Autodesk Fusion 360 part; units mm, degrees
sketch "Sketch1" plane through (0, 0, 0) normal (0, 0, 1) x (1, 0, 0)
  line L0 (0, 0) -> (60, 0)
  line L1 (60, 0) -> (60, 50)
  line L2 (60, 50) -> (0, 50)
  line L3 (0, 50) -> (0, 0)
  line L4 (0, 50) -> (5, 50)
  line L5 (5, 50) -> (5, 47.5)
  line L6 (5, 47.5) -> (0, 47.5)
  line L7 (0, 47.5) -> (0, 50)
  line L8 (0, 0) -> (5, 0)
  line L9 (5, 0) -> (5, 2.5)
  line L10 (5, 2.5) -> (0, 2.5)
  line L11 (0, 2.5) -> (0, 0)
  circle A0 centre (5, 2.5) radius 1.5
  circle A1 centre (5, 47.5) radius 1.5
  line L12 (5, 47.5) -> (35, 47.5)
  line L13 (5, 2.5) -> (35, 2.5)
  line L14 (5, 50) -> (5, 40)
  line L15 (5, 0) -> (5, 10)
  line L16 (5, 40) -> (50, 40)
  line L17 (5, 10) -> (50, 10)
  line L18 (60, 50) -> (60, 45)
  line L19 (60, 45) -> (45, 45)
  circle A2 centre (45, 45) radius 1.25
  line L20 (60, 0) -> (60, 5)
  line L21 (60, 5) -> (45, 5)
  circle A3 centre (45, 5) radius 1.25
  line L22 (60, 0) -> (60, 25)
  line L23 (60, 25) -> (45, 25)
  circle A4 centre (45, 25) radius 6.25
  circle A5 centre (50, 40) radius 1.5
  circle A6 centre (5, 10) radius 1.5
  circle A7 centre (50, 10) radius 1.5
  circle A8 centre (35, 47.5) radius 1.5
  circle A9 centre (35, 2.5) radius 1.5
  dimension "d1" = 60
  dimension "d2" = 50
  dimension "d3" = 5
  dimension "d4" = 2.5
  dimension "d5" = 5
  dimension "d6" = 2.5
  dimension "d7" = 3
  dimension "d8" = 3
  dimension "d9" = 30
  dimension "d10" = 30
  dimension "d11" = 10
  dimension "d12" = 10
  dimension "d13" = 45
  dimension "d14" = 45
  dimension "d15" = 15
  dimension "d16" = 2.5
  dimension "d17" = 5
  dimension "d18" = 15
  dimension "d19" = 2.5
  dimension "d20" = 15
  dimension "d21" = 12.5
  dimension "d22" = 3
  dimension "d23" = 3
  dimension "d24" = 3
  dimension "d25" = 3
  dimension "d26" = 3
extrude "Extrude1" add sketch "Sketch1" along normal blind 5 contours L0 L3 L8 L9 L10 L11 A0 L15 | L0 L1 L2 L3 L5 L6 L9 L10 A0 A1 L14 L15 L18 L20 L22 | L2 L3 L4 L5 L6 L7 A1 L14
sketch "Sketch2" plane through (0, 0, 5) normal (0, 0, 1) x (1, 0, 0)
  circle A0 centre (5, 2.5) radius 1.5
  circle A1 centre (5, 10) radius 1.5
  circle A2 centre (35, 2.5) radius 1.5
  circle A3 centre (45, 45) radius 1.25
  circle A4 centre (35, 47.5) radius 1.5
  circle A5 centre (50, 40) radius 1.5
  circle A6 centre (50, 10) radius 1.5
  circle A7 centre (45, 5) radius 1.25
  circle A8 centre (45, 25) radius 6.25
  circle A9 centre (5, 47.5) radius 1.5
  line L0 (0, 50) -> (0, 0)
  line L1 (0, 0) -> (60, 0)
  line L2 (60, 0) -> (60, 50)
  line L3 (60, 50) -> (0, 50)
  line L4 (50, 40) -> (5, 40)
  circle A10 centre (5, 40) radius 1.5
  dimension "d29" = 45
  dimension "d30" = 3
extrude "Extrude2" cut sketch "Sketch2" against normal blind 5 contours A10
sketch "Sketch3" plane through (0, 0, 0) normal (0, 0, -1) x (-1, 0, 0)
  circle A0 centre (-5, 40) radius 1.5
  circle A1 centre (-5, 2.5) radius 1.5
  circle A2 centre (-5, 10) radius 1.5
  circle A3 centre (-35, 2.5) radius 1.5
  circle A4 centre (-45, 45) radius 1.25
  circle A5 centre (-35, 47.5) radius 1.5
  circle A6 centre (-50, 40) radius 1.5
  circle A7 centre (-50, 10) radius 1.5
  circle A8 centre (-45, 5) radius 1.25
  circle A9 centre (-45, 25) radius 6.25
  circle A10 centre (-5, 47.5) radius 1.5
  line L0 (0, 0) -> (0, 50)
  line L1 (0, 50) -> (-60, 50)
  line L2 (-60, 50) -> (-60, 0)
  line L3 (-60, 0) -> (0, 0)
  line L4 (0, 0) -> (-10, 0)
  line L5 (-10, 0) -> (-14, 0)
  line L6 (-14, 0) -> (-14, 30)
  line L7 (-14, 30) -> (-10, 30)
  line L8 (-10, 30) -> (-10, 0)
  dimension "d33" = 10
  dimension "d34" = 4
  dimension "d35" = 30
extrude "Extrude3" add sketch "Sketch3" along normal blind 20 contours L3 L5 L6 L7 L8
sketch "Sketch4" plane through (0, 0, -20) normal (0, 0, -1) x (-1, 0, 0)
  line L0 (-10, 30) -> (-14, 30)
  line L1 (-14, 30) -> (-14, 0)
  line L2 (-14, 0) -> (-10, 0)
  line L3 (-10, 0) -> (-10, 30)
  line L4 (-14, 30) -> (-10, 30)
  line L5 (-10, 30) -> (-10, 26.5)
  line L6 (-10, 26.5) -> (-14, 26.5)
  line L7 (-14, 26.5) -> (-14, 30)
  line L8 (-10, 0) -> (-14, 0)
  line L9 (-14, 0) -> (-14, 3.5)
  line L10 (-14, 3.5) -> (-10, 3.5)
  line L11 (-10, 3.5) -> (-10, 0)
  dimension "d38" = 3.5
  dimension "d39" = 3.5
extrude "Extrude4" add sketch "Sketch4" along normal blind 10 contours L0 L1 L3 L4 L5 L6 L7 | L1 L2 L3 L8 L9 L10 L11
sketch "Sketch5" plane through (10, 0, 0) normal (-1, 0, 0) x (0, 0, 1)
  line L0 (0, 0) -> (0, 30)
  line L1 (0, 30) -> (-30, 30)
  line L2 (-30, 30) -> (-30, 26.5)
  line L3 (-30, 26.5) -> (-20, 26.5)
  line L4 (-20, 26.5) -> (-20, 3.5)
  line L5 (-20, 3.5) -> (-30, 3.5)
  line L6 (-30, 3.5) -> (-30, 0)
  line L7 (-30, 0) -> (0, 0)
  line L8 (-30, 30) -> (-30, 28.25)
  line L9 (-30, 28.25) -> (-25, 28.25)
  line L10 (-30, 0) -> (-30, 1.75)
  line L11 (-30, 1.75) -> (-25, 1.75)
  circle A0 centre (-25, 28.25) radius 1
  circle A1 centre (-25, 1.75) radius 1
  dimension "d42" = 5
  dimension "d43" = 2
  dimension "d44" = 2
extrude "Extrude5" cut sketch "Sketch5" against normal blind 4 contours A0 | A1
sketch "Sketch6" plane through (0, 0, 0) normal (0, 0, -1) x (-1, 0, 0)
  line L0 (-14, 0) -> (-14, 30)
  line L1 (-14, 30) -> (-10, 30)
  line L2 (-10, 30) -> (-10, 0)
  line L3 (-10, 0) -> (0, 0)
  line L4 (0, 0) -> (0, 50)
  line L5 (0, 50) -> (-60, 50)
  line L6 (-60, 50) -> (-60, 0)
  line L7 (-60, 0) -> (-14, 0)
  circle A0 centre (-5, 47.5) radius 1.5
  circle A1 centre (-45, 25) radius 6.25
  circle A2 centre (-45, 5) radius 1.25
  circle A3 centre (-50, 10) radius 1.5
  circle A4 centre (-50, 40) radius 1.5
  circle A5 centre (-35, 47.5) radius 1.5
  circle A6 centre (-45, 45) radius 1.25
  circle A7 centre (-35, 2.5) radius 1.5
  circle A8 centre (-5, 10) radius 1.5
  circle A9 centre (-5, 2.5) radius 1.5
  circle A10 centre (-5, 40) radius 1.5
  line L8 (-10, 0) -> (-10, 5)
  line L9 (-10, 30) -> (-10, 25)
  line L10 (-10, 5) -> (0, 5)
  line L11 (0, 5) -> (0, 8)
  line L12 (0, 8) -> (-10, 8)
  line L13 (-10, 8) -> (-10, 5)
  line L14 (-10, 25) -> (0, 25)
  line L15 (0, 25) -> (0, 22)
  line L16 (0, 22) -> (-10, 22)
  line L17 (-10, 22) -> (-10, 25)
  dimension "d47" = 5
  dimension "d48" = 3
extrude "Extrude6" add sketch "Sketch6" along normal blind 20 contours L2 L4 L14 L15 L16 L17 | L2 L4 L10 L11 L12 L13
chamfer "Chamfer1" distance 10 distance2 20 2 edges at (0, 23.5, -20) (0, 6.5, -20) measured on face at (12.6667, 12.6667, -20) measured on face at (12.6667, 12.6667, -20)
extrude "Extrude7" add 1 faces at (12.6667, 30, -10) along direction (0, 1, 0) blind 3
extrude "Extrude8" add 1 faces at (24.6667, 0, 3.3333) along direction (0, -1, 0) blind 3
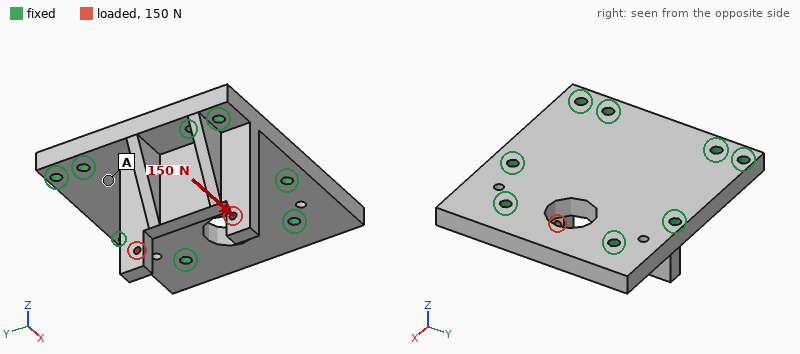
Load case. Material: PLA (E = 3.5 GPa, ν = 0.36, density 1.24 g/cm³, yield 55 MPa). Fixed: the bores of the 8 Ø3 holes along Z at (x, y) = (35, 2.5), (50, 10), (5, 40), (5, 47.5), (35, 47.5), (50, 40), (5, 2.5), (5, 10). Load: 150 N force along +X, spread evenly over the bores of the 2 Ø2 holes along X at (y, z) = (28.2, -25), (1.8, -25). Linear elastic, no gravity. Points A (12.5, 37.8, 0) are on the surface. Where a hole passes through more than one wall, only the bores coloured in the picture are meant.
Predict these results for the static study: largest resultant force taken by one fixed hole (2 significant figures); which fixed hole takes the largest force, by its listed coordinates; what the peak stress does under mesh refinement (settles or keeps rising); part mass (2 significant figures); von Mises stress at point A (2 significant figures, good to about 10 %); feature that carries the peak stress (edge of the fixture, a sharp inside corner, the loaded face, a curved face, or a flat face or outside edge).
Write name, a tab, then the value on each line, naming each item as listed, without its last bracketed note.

largest resultant force taken by one fixed hole	110 N
which fixed hole takes the largest force, by its listed coordinates	(5, 10)
what the peak stress does under mesh refinement	keeps rising
part mass	23 g
von Mises stress at point A	2.9 MPa
feature that carries the peak stress	edge of the fixture
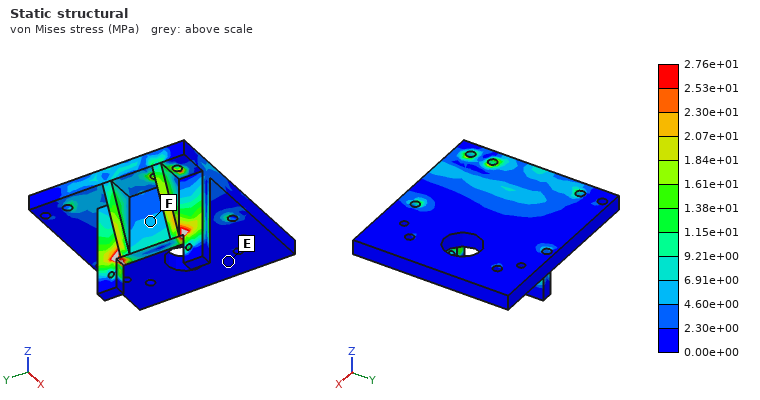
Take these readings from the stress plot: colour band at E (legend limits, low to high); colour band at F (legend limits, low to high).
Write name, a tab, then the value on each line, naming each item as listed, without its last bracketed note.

colour band at E	0.00e+00 to 2.30e+00 MPa
colour band at F	4.60e+00 to 6.91e+00 MPa
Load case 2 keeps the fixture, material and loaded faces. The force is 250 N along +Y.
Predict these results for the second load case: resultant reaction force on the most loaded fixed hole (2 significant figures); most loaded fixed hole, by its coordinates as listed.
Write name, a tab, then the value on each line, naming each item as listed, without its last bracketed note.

resultant reaction force on the most loaded fixed hole	200 N
most loaded fixed hole, by its coordinates as listed	(5, 2.5)
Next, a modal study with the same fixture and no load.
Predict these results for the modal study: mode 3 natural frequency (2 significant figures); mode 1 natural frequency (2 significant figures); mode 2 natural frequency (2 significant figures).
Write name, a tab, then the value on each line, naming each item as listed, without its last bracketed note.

mode 3 natural frequency	4000 Hz
mode 1 natural frequency	2300 Hz
mode 2 natural frequency	2700 Hz
